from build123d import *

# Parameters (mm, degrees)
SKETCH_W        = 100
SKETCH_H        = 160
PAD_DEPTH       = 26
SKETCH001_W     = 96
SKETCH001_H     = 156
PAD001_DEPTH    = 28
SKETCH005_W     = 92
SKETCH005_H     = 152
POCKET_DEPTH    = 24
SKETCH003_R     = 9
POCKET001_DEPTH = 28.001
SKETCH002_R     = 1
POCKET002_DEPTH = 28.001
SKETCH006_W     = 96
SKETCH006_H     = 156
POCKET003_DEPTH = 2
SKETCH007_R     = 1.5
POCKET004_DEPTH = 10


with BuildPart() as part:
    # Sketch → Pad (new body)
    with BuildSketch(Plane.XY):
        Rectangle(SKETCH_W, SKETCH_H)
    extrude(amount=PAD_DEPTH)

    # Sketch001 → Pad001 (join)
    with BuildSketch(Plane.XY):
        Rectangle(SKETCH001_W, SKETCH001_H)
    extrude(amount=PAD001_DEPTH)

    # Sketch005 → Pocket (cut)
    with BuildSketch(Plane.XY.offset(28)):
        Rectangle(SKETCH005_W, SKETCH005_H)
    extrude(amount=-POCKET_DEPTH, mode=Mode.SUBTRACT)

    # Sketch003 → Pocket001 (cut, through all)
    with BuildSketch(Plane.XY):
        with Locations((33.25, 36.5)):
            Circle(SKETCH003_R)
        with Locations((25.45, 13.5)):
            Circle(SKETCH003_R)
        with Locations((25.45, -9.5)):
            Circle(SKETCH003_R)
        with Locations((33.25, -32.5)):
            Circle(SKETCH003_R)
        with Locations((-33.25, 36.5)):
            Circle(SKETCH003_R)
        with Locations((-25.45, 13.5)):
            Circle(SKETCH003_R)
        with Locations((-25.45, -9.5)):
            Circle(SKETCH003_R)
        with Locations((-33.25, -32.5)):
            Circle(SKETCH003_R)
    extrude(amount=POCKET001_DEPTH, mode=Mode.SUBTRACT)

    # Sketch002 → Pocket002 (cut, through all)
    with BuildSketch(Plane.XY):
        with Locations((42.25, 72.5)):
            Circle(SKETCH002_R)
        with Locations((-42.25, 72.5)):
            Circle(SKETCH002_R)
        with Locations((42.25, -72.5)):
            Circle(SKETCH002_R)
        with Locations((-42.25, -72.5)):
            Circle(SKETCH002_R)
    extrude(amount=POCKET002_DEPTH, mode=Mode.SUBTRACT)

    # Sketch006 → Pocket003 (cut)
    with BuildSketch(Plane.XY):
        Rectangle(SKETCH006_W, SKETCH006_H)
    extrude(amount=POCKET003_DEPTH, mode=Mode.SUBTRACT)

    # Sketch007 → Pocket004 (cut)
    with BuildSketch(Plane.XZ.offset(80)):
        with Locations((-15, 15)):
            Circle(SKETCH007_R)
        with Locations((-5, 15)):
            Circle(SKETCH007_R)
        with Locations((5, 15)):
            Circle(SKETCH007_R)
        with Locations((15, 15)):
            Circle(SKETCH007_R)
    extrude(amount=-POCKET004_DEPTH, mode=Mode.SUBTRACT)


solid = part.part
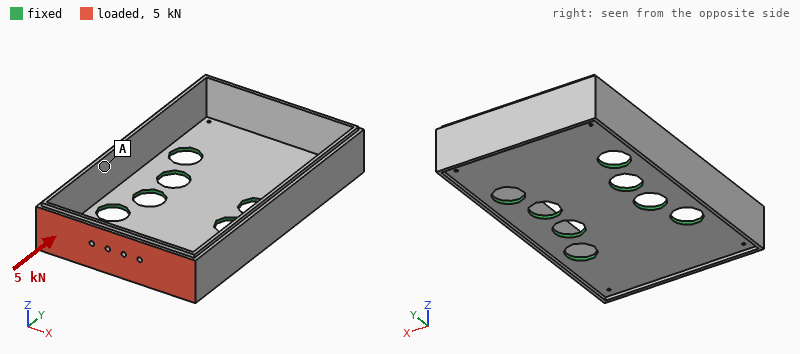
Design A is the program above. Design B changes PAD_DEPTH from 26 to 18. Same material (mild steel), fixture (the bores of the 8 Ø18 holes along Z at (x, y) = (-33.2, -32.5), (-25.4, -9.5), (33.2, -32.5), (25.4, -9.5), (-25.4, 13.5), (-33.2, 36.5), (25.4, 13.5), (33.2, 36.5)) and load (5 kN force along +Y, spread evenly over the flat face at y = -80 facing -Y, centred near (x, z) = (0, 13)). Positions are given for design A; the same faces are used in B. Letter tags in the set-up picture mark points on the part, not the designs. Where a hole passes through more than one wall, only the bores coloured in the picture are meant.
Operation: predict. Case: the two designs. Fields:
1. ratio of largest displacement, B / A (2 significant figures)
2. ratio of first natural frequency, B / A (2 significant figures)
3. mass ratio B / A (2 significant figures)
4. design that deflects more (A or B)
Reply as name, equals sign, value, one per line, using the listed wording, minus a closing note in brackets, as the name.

ratio of largest displacement, B / A = 0.82
ratio of first natural frequency, B / A = 0.98
mass ratio B / A = 0.89
design that deflects more = A
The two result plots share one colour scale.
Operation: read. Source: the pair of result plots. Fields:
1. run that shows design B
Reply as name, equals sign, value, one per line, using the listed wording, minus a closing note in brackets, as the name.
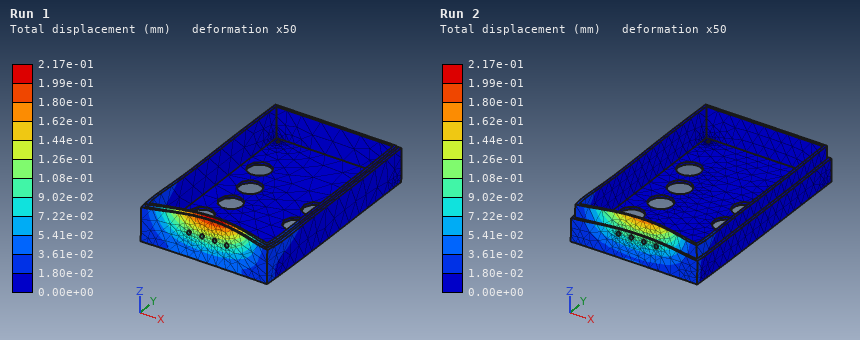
run that shows design B = Run 2
